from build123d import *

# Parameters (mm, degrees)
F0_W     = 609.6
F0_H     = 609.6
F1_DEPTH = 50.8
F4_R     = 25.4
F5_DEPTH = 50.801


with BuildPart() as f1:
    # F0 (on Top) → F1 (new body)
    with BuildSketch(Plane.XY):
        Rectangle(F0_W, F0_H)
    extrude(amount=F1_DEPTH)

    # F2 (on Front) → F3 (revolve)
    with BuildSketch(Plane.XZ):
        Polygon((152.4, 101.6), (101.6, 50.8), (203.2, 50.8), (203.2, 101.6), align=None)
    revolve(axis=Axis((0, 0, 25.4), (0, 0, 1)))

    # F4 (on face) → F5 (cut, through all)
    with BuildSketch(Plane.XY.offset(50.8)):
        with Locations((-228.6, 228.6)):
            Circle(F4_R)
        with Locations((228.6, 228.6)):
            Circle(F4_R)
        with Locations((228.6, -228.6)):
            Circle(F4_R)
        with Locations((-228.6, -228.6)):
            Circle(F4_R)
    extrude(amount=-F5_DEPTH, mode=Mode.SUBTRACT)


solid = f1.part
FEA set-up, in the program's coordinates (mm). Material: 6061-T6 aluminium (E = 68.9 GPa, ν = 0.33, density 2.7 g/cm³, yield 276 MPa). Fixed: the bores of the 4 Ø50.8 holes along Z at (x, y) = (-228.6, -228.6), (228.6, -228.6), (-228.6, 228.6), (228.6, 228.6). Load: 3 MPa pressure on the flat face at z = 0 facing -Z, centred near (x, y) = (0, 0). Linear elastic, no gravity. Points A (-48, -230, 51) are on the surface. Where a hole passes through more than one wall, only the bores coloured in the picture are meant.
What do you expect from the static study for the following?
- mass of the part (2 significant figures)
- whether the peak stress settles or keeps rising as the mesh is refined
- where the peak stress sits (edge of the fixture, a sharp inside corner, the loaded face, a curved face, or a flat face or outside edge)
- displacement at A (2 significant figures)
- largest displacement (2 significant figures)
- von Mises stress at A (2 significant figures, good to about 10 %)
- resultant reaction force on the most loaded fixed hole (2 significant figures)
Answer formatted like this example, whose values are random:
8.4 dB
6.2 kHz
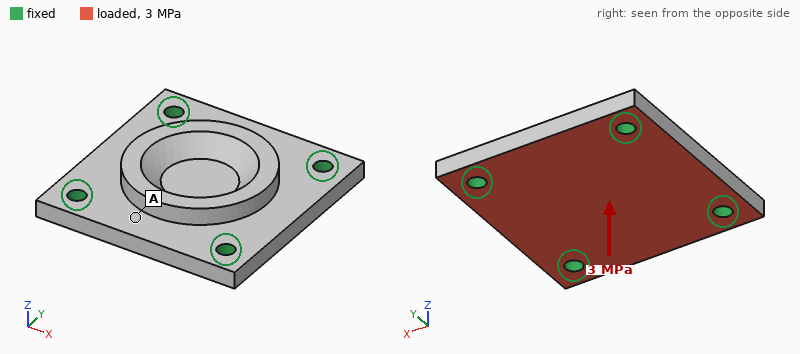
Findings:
61 kg
keeps rising
edge of the fixture
0.42 mm
0.64 mm
40 MPa
280 kN
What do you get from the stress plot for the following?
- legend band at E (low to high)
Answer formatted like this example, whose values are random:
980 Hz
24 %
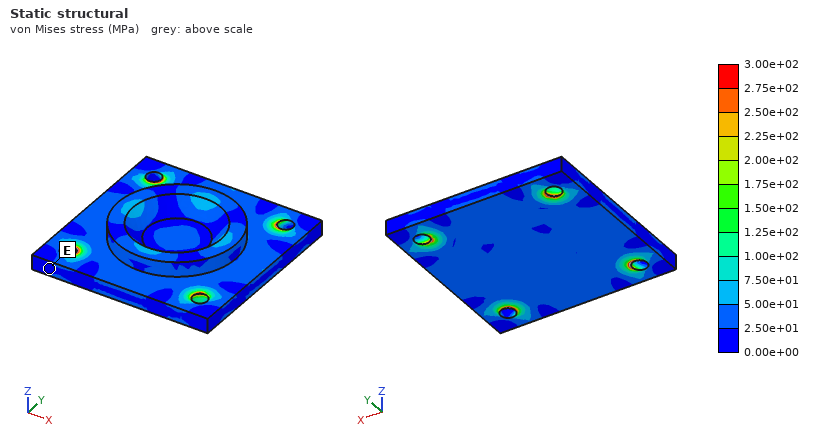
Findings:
0.00e+00 to 2.50e+01 MPa
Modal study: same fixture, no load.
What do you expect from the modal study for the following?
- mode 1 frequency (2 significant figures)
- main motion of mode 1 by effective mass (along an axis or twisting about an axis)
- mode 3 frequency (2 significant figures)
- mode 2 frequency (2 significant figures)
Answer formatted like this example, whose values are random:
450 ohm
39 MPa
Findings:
950 Hz
along Z
1400 Hz
1400 Hz
